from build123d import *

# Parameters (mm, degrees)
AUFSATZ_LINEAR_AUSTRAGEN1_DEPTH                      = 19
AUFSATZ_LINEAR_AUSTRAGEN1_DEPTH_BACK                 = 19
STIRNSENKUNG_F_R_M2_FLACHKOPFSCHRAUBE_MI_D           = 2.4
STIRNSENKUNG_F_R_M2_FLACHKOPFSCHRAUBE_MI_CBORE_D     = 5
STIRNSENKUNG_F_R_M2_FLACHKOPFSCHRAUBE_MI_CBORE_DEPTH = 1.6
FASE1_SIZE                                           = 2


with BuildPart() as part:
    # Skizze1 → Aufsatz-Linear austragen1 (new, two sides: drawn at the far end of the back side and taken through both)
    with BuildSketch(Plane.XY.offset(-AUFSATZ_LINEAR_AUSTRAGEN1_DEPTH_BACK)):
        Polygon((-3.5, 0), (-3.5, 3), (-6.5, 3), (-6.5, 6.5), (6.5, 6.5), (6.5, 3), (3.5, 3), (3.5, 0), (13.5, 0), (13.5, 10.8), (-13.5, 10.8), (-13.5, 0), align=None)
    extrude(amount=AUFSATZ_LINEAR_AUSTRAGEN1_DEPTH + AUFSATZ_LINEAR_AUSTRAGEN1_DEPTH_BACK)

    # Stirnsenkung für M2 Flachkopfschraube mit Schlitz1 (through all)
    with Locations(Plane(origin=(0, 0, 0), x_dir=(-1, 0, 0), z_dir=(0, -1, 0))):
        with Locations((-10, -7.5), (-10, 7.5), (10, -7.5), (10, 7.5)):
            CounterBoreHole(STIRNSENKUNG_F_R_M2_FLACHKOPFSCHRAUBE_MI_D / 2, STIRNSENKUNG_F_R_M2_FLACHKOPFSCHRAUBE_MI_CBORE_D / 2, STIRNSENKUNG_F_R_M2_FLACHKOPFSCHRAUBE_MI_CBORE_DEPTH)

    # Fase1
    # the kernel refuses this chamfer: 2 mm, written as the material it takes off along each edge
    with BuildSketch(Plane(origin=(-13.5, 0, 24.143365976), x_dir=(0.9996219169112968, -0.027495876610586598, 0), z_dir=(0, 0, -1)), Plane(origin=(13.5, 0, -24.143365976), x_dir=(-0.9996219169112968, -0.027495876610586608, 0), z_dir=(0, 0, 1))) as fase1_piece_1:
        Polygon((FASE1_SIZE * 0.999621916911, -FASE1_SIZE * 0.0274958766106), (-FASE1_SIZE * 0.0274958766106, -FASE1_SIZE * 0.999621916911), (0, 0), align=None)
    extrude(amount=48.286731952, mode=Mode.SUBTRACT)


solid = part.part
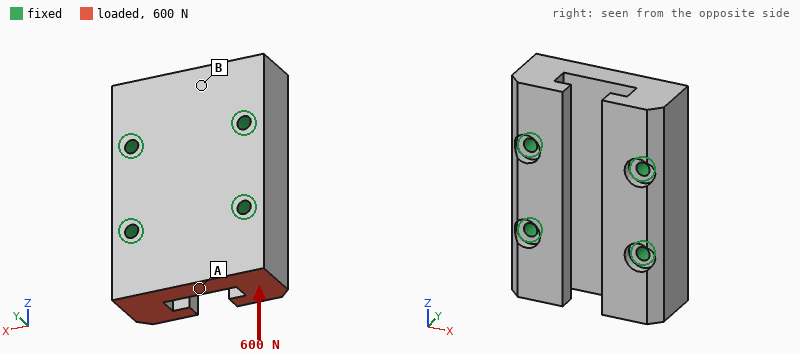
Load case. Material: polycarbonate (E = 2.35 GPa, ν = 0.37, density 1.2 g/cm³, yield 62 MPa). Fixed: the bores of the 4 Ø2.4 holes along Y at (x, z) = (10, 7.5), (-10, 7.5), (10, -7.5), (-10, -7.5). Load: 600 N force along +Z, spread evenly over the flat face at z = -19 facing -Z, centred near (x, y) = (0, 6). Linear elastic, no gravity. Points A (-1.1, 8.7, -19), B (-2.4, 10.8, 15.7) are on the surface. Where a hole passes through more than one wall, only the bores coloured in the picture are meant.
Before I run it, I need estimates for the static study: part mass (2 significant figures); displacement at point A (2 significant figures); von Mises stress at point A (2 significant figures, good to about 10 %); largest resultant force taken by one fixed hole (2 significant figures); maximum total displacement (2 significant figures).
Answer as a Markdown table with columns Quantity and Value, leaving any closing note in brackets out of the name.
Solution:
| Quantity | Value |
|---|---|
| part mass | 9.7 g |
| displacement at point A | 18 µm |
| von Mises stress at point A | 2.3 MPa |
| largest resultant force taken by one fixed hole | 260 N |
| maximum total displacement | 20 µm |
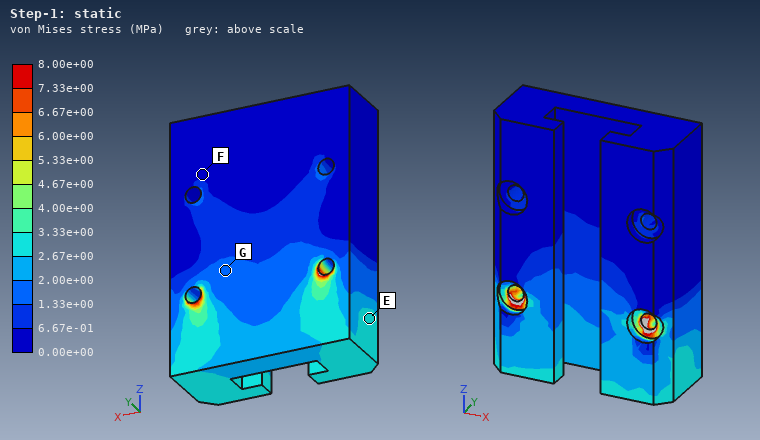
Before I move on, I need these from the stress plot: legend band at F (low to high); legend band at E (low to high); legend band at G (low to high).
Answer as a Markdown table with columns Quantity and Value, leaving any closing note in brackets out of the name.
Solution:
| Quantity | Value |
|---|---|
| legend band at F | 0.00e+00 to 6.67e-01 MPa |
| legend band at E | 2.67e+00 to 3.33e+00 MPa |
| legend band at G | 1.33e+00 to 2.00e+00 MPa |
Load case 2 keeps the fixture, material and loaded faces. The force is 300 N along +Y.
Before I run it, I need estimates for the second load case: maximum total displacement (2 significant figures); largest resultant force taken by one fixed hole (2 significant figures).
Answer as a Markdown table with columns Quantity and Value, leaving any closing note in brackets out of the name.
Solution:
| Quantity | Value |
|---|---|
| maximum total displacement | 0.12 mm |
| largest resultant force taken by one fixed hole | 170 N |
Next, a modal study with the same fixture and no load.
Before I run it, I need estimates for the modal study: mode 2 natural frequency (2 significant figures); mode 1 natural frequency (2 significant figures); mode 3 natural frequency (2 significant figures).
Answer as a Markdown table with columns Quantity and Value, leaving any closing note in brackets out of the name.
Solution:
| Quantity | Value |
|---|---|
| mode 2 natural frequency | 8800 Hz |
| mode 1 natural frequency | 8600 Hz |
| mode 3 natural frequency | 11 kHz |
